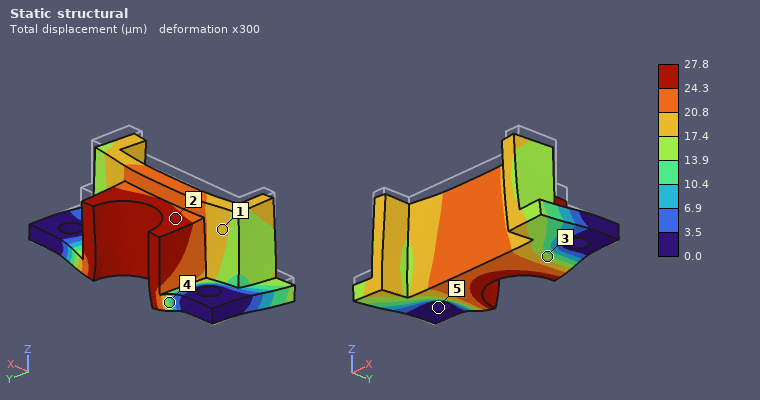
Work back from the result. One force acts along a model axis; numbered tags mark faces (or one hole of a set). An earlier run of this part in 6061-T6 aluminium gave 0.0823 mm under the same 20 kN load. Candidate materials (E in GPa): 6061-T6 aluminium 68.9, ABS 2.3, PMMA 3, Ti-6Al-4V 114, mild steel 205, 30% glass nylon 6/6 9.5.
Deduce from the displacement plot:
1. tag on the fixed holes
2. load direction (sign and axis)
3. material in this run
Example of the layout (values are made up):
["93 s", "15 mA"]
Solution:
["5", "-Z", "mild steel"]
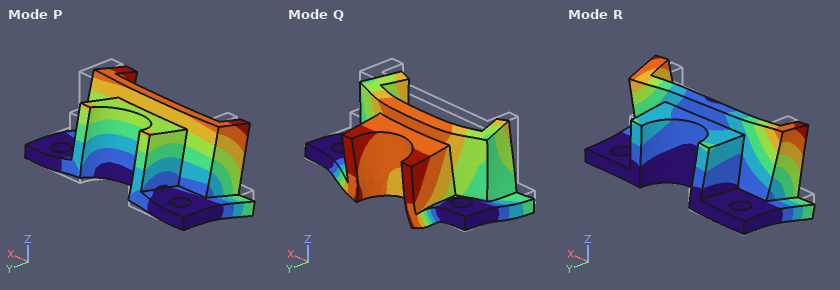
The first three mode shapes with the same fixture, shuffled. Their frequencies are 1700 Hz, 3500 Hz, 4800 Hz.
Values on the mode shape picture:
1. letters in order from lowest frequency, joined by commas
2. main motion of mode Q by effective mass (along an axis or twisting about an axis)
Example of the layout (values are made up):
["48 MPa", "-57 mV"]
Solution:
["P, R, Q", "along Z"]
